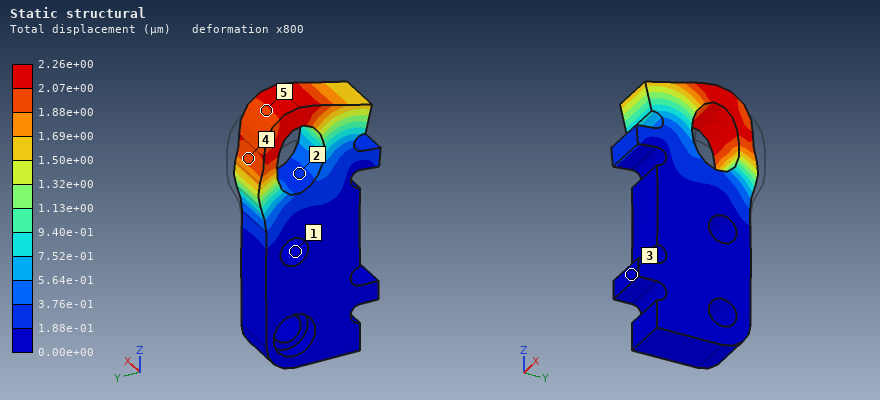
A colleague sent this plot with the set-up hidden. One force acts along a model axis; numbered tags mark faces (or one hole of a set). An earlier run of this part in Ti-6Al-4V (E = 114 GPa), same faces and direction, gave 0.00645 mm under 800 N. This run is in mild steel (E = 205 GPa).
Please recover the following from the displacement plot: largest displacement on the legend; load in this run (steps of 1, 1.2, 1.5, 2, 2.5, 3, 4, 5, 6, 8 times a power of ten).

2.26e+00 µm
500 N
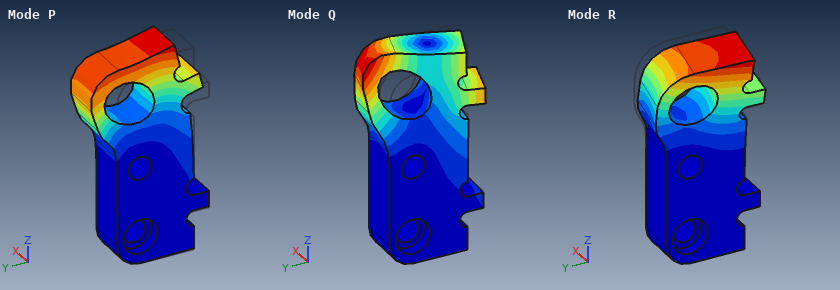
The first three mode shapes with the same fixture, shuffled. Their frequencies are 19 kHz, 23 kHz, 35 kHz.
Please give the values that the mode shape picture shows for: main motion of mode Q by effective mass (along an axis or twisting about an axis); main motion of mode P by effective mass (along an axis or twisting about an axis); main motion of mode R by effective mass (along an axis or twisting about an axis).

twisting about Z
along Y
along X
